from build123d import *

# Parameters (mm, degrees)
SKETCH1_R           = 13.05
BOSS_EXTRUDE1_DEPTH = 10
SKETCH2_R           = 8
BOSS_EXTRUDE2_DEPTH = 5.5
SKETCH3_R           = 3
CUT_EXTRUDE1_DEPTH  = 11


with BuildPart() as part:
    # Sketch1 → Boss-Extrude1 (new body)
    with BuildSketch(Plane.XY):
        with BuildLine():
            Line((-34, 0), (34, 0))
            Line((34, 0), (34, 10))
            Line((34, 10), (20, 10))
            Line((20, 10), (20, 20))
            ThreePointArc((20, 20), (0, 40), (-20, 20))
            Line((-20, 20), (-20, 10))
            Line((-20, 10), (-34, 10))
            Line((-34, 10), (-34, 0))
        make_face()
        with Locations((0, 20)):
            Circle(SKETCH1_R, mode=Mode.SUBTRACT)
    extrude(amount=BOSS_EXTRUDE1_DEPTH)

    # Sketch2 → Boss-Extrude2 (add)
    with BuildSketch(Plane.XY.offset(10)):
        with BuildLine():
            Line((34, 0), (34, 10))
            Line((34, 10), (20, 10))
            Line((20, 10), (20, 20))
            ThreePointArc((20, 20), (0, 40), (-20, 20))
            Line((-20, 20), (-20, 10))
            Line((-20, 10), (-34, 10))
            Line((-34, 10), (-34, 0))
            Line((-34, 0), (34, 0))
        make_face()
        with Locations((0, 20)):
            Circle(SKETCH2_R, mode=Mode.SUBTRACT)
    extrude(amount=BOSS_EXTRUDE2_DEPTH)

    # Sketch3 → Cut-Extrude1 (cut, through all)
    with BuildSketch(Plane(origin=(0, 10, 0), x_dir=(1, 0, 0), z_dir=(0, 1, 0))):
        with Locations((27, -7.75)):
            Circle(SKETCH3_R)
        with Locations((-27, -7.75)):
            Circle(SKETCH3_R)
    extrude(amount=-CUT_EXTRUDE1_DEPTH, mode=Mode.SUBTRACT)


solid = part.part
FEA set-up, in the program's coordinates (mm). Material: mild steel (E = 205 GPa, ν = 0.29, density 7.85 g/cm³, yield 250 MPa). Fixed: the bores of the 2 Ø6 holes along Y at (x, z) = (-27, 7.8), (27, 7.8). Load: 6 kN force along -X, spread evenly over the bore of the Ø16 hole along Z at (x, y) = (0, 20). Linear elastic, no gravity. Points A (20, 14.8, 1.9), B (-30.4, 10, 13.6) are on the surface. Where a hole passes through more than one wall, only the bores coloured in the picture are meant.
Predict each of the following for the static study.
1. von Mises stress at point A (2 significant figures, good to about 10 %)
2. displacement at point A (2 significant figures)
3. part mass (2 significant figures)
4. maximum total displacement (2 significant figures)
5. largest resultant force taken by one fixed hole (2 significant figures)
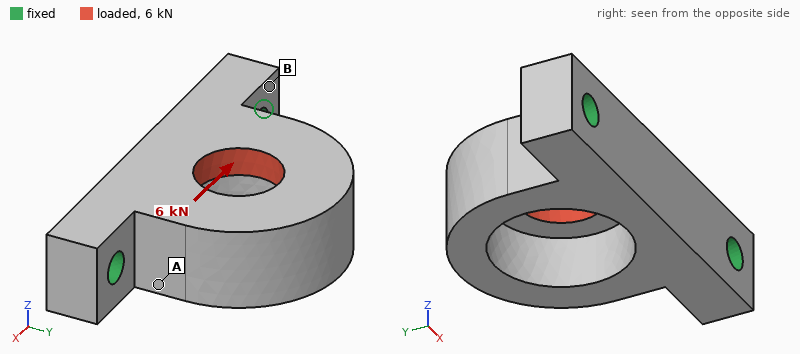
35 MPa
3.8 µm
150 g
12 µm
3.6 kN
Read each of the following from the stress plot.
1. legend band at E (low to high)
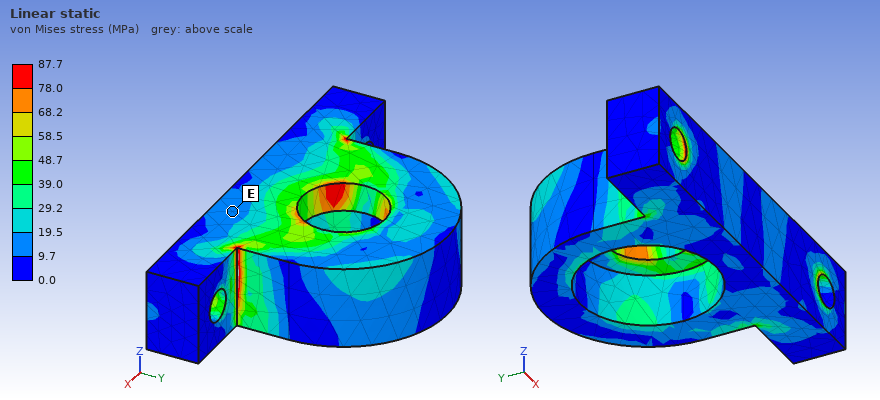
9.7 to 19.5 MPa
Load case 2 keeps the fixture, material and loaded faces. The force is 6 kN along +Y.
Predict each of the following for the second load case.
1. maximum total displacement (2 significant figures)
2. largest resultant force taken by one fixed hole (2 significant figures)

28 µm
3.1 kN
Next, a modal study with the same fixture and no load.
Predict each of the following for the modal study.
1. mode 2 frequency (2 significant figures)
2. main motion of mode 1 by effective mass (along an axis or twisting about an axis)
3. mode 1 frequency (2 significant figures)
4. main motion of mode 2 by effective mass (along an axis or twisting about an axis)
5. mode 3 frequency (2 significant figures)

11 kHz
along Z
5200 Hz
along X
15 kHz
